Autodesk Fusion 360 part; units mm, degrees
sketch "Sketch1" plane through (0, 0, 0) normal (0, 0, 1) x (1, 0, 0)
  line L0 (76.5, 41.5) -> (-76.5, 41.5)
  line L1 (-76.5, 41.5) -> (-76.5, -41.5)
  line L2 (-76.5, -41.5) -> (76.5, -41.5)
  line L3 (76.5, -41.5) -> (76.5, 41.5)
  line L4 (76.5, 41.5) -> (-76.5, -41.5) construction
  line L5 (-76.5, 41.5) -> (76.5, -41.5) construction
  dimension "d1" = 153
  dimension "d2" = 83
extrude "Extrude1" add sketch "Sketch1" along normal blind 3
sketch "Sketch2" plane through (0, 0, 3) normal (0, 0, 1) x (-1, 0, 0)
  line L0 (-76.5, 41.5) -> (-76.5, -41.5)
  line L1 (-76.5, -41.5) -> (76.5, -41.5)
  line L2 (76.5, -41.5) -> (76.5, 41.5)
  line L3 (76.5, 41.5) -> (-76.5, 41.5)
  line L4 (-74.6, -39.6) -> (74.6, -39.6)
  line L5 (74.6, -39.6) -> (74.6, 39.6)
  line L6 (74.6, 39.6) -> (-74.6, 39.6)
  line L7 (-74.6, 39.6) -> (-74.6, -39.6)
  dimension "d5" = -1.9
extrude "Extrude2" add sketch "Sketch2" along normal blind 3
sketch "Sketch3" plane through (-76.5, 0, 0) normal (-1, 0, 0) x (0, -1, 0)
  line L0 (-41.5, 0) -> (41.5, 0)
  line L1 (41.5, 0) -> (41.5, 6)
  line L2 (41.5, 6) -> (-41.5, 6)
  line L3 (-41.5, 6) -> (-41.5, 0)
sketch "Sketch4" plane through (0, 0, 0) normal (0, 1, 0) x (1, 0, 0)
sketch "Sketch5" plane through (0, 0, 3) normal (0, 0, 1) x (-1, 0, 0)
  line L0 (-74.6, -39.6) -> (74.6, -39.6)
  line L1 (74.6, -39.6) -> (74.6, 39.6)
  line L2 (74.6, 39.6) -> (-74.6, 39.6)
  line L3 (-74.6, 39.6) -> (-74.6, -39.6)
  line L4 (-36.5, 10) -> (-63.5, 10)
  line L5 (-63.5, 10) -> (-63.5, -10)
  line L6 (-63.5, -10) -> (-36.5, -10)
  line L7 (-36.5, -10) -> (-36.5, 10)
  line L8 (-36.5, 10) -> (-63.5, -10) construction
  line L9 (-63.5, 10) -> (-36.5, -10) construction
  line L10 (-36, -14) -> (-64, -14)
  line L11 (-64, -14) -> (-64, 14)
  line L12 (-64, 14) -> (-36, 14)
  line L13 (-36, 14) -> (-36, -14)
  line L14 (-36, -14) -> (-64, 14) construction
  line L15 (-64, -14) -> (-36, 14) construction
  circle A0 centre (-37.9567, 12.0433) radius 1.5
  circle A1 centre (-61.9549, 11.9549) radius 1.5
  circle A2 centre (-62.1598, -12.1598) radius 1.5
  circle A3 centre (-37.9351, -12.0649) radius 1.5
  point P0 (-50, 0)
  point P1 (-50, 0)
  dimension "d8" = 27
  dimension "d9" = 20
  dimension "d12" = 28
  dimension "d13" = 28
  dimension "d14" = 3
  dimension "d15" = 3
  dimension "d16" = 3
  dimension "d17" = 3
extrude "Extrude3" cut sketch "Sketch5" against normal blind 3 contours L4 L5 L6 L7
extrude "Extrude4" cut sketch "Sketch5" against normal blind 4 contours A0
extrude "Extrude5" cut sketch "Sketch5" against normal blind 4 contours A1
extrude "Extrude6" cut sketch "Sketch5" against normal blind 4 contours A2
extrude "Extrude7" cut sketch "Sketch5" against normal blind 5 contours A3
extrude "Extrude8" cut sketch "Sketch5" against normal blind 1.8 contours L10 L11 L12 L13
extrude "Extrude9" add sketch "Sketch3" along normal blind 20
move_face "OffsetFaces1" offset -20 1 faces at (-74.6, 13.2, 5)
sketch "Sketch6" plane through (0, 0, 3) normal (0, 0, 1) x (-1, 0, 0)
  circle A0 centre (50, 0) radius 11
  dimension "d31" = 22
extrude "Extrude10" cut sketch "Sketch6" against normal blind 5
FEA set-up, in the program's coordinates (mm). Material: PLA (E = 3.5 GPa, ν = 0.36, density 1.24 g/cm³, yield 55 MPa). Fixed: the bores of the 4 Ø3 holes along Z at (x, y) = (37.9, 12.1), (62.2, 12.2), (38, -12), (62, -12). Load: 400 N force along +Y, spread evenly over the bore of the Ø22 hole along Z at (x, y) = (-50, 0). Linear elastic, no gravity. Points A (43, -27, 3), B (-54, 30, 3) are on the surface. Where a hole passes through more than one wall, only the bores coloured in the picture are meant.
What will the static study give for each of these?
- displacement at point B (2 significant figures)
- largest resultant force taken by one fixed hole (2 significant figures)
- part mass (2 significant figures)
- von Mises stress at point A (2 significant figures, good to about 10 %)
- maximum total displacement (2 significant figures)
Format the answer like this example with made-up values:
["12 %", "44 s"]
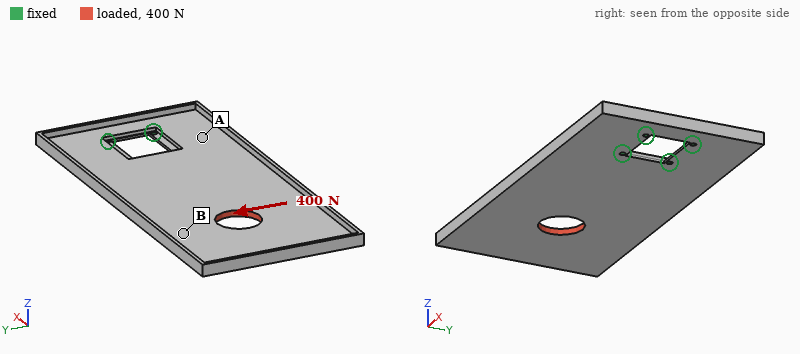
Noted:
["0.88 mm", "690 N", "53 g", "8.9 MPa", "1.3 mm"]
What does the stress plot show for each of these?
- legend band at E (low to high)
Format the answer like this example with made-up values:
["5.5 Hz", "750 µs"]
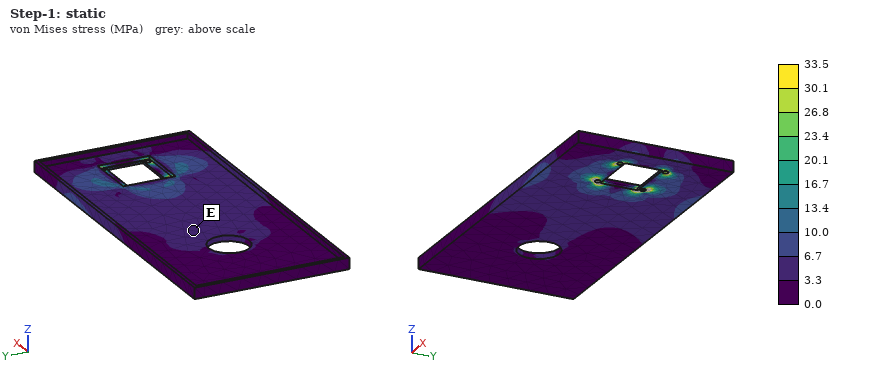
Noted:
["3.3 to 6.7 MPa"]
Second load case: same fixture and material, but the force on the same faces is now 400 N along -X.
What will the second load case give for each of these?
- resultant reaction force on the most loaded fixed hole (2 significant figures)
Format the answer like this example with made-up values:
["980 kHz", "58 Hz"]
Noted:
["150 N"]
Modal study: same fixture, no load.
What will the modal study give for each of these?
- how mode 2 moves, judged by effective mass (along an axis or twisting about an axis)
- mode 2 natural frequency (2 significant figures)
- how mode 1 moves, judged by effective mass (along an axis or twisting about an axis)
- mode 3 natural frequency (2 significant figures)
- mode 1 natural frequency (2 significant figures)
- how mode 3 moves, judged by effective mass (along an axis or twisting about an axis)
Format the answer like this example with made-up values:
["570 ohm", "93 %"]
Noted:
["twisting about X", "130 Hz", "along Z", "270 Hz", "45 Hz", "along Z"]
